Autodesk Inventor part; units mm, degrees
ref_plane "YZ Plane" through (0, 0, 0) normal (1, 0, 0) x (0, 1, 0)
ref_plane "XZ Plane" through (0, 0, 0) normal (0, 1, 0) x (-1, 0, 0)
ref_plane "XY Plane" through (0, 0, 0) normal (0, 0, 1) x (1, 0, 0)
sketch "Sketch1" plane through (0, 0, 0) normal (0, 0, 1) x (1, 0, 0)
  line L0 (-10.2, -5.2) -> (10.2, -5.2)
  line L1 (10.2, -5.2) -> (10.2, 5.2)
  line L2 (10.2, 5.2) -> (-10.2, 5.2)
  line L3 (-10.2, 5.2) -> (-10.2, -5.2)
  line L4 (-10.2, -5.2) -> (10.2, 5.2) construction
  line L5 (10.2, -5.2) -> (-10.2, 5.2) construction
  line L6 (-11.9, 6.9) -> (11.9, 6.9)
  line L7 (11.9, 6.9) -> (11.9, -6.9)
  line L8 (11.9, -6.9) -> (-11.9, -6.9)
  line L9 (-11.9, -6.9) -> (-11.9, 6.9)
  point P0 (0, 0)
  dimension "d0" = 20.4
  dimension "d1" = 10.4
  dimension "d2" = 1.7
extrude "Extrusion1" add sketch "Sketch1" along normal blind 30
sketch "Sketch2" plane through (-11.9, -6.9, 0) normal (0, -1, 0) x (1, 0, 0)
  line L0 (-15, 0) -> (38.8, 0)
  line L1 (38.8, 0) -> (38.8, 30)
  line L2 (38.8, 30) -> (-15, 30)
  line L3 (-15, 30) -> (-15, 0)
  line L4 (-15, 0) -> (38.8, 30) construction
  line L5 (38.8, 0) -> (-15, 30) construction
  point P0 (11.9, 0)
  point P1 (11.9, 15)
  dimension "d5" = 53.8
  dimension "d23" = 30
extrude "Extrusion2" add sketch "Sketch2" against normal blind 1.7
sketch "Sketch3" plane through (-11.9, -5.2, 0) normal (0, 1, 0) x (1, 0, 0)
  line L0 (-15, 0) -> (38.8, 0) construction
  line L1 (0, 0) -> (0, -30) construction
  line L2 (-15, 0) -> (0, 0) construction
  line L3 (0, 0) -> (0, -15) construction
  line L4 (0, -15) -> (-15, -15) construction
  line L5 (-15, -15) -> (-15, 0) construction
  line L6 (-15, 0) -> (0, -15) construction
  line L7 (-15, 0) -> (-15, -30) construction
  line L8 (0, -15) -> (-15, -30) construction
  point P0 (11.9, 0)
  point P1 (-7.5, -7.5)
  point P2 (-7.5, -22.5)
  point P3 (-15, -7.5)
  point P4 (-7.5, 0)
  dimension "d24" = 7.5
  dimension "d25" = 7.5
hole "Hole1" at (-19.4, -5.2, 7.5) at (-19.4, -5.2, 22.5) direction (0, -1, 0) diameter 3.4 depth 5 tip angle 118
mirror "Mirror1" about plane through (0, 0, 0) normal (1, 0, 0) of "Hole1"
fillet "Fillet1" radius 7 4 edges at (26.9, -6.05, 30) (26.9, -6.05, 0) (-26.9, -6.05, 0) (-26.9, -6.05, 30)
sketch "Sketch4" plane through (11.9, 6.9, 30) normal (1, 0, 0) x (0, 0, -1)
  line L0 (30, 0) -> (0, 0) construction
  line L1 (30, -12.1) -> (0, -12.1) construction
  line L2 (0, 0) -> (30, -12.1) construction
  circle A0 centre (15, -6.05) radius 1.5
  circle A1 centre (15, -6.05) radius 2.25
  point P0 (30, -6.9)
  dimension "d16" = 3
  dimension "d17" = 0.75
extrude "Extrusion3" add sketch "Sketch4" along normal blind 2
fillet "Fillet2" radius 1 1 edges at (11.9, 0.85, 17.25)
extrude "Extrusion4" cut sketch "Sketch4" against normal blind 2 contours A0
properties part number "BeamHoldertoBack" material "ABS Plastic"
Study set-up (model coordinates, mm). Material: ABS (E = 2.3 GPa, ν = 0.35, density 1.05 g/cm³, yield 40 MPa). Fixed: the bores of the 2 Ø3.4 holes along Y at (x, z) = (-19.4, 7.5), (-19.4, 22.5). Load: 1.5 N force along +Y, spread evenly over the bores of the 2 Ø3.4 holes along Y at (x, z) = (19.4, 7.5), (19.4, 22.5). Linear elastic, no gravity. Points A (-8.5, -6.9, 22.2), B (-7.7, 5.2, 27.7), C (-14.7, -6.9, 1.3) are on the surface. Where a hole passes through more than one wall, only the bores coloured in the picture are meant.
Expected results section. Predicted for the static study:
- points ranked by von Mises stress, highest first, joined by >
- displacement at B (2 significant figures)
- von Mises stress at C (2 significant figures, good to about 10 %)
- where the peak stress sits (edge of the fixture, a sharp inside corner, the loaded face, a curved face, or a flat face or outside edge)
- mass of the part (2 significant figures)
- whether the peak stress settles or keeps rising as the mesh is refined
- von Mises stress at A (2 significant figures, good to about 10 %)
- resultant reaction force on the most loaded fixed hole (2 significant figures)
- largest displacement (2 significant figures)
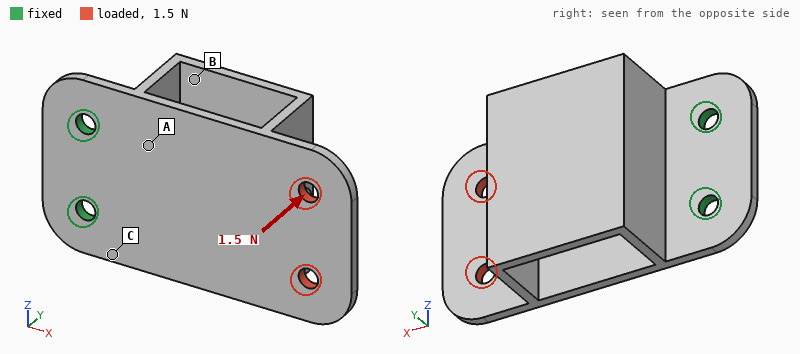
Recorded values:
C > A > B
0.21 mm
3.0 MPa
edge of the fixture
5.1 g
keeps rising
1.1 MPa
0.75 N
0.72 mm
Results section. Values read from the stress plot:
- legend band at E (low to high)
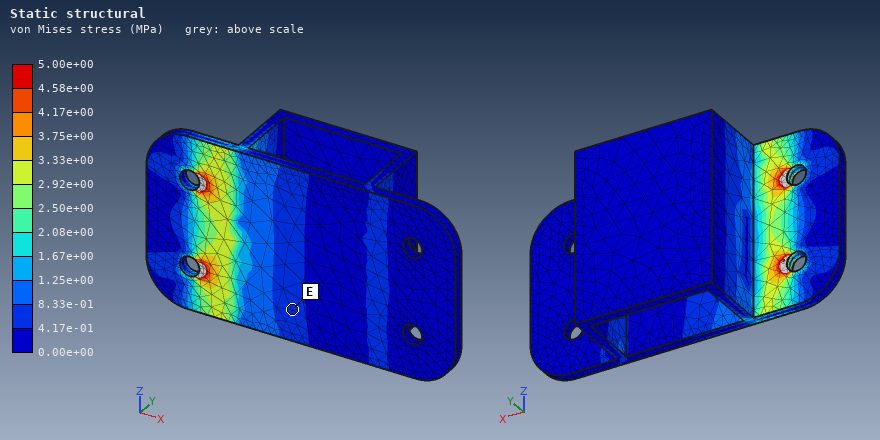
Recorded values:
4.17e-01 to 8.33e-01 MPa
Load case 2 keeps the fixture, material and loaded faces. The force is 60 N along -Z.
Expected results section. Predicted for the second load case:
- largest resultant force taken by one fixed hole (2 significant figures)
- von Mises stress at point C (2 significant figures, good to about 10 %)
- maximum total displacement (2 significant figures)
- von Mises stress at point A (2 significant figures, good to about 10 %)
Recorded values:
140 N
4.5 MPa
0.31 mm
4.7 MPa
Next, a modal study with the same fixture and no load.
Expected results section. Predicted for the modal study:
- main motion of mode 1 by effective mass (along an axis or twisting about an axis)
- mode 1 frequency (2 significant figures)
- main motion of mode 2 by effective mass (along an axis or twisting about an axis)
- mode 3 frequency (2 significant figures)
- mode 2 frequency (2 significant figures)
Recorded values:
along Y
190 Hz
along Z
1600 Hz
960 Hz
